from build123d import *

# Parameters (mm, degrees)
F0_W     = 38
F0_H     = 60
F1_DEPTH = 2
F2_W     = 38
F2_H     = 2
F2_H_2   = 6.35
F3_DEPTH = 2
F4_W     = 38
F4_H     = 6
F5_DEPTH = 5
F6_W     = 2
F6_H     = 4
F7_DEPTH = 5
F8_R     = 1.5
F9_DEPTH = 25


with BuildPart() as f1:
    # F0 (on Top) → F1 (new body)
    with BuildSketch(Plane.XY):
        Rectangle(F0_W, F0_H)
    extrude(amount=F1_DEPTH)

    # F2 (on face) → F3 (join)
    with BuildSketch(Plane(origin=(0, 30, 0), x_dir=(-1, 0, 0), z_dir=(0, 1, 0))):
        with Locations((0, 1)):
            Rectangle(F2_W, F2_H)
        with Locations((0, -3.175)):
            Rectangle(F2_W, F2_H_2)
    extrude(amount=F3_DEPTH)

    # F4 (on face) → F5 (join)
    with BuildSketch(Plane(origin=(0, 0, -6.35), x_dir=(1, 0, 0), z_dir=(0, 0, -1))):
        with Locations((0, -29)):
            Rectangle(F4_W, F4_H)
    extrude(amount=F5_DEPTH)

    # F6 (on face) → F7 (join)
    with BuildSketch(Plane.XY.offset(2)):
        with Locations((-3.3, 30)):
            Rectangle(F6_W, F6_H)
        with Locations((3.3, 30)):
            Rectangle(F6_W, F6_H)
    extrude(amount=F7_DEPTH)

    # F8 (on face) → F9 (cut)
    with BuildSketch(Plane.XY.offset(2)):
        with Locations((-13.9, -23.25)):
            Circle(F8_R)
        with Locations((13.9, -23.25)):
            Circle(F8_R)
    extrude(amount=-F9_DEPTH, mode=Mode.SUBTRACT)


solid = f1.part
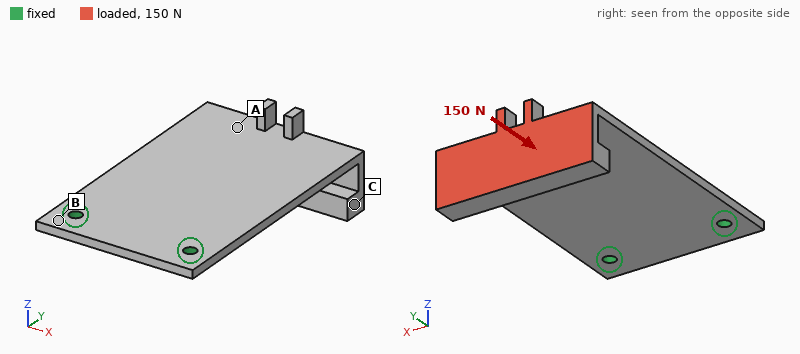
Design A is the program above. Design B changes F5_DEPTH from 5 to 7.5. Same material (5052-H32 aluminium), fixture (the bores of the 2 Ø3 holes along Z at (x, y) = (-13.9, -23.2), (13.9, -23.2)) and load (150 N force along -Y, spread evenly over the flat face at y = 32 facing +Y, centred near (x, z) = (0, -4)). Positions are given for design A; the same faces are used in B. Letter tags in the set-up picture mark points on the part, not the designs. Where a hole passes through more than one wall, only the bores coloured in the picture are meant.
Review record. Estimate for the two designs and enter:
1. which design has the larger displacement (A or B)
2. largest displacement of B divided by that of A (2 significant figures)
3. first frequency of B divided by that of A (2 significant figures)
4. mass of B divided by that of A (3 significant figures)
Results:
B
1.3
0.91
1.09
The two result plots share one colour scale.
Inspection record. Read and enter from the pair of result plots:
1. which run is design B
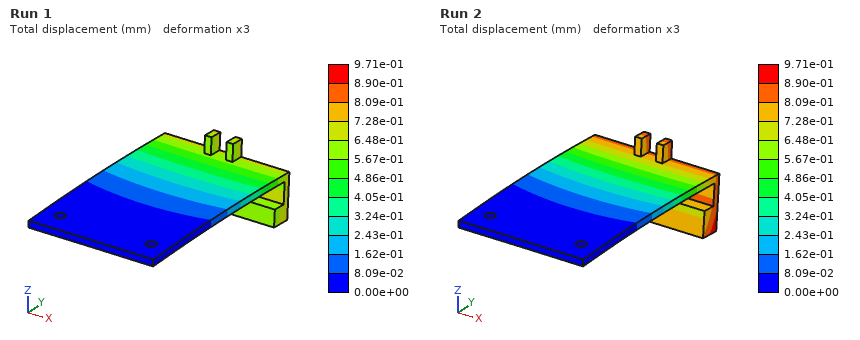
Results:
Run 2
